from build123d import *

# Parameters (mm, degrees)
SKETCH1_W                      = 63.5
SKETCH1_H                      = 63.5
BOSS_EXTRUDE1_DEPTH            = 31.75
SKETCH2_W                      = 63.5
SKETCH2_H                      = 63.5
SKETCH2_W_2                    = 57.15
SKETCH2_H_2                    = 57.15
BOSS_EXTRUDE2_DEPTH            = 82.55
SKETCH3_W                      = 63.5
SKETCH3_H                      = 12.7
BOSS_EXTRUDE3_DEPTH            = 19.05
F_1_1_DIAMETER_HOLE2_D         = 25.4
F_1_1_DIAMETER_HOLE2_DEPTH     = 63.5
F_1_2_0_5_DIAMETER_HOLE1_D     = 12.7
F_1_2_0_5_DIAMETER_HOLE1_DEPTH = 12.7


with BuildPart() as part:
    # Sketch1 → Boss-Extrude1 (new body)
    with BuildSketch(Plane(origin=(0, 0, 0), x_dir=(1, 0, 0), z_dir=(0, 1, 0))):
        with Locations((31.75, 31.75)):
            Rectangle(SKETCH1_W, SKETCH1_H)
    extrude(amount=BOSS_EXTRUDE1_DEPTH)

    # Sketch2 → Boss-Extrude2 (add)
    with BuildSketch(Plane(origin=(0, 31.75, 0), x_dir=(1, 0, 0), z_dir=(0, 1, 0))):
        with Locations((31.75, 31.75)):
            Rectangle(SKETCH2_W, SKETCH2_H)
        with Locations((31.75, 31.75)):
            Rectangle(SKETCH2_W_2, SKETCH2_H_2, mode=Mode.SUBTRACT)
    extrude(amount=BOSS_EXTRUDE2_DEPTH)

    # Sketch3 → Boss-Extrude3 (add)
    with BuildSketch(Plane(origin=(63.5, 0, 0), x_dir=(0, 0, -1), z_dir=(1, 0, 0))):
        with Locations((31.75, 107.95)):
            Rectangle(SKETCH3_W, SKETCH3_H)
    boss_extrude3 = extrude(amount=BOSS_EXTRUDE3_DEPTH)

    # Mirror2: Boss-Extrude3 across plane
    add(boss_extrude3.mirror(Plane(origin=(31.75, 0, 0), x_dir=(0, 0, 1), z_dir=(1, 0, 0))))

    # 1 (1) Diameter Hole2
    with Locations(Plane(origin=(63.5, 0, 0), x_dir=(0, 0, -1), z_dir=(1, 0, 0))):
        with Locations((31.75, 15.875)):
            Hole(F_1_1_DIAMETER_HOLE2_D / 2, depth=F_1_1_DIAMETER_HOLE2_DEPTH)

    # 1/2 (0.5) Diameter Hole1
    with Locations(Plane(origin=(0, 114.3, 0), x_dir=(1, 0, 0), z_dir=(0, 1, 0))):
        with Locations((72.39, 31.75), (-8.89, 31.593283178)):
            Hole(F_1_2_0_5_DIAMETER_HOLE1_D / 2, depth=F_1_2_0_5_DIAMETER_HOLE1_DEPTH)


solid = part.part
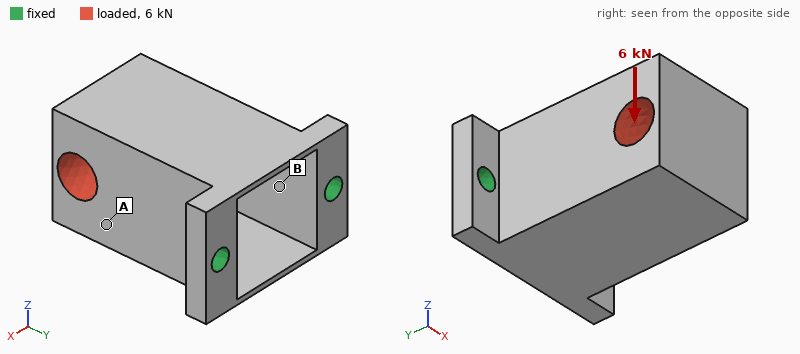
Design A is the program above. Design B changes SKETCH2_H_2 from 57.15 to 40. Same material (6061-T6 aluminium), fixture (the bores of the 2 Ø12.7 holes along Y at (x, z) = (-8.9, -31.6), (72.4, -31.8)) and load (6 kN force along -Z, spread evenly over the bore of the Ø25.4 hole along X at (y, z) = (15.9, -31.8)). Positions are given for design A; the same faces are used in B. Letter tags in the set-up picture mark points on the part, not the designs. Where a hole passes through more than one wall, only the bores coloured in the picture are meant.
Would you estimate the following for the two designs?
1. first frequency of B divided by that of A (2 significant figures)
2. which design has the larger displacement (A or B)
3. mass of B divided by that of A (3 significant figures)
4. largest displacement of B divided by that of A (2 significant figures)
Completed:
0.98
A
1.43
0.88
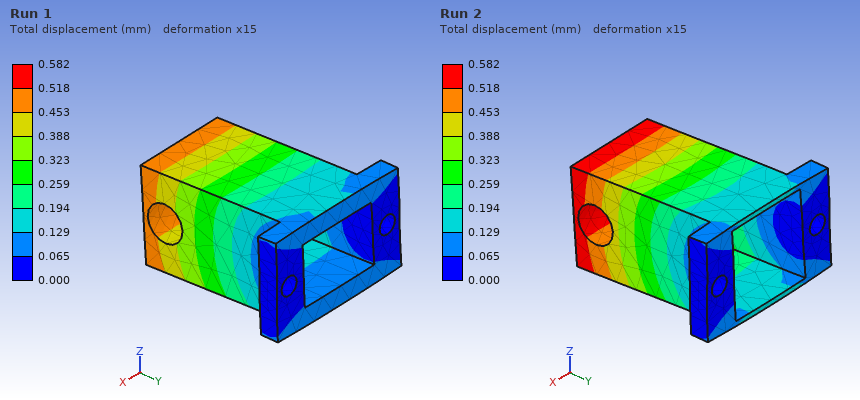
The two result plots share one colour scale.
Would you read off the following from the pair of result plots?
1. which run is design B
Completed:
Run 1
